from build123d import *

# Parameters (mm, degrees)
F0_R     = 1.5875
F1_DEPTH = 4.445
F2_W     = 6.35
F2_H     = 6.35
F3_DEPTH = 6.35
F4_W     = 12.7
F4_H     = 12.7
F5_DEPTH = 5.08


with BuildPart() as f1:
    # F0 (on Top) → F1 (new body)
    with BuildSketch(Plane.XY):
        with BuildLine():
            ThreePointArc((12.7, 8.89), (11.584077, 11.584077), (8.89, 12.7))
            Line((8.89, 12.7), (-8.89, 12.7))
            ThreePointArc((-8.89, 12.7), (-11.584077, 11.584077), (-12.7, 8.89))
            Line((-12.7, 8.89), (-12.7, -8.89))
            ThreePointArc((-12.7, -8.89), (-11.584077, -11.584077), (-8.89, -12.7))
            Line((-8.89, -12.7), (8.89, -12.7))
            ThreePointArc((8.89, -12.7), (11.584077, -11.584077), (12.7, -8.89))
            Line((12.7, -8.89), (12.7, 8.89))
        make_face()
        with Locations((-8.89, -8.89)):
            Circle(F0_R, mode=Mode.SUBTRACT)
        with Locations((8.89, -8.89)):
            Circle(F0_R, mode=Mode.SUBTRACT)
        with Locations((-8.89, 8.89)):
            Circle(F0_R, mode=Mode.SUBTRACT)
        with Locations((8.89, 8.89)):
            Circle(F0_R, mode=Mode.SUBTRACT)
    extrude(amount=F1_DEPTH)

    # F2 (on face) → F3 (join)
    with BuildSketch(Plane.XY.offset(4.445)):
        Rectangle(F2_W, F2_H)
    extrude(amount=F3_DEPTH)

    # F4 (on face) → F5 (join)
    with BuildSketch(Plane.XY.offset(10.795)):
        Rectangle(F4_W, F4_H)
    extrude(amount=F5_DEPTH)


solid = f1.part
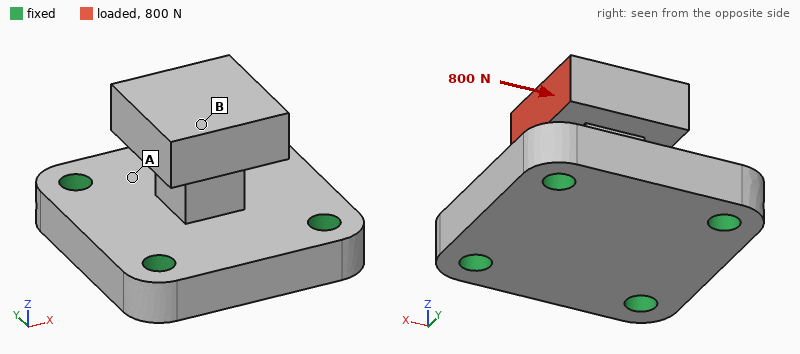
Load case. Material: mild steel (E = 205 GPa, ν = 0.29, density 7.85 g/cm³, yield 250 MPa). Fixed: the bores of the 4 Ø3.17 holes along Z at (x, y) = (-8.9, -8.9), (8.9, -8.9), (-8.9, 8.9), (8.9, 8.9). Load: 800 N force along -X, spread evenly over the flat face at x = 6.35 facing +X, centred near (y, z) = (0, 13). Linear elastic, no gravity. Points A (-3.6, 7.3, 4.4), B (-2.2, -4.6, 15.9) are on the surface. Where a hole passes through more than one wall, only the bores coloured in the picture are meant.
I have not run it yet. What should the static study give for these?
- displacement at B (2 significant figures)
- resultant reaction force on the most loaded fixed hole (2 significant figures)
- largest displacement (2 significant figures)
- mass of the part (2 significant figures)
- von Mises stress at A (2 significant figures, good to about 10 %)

21 µm
370 N
25 µm
29 g
21 MPa
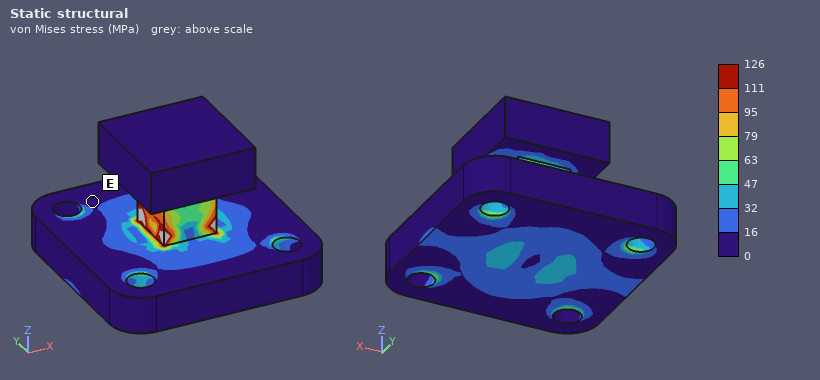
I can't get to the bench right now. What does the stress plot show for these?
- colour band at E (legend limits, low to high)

0 to 16 MPa
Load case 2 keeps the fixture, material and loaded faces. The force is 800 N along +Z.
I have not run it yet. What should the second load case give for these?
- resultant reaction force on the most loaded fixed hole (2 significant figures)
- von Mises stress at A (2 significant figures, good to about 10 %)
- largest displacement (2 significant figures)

370 N
11 MPa
24 µm
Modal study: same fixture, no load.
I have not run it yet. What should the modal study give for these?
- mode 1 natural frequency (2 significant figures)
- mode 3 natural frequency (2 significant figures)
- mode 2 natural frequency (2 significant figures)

12 kHz
18 kHz
12 kHz
